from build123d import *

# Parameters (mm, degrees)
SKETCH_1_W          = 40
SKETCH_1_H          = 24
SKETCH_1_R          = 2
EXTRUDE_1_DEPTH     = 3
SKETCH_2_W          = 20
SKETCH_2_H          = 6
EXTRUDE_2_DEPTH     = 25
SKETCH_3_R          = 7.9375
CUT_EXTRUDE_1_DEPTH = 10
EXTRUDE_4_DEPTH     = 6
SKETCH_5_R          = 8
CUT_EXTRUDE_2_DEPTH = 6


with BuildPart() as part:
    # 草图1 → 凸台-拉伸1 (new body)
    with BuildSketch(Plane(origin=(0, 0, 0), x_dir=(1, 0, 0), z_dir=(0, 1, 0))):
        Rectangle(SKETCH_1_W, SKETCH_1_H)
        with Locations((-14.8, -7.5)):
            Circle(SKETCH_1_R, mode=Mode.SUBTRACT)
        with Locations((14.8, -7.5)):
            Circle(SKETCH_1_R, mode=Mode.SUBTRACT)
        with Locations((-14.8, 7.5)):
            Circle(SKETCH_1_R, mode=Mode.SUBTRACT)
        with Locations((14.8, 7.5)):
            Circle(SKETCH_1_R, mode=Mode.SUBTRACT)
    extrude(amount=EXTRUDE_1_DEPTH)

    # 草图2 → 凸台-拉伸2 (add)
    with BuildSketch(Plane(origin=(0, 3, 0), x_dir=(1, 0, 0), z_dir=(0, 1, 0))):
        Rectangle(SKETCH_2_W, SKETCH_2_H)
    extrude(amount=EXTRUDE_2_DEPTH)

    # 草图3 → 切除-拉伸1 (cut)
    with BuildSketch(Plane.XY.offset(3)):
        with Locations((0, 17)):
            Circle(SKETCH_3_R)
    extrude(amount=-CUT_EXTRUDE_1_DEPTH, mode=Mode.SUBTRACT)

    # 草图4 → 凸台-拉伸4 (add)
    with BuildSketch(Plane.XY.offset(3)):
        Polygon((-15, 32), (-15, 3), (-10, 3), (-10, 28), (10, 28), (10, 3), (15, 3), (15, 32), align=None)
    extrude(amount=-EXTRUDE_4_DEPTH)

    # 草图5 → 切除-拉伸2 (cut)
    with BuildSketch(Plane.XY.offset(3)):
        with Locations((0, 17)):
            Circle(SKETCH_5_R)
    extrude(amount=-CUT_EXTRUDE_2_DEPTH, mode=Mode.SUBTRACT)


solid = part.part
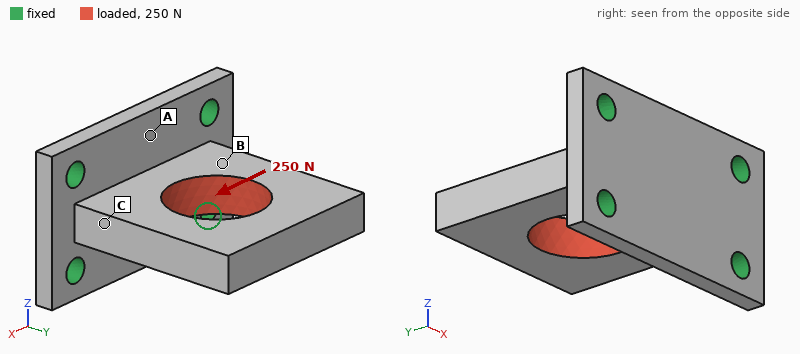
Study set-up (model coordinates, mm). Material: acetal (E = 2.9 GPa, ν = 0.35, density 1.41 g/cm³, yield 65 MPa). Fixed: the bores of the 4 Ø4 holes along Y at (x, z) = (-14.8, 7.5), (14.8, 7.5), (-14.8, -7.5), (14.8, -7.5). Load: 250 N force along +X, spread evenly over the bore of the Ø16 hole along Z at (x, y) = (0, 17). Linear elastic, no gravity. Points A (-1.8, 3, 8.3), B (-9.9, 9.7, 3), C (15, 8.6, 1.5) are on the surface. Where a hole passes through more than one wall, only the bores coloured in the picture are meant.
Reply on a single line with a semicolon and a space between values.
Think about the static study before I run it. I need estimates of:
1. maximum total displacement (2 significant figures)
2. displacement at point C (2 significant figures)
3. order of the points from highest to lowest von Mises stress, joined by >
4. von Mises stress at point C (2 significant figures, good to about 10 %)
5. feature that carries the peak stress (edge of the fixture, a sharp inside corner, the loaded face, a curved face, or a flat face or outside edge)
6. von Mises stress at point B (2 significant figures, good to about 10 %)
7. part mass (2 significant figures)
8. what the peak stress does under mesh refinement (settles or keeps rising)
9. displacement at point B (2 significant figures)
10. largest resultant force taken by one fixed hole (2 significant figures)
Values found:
0.16 mm; 0.048 mm; C > B > A; 6.1 MPa; edge of the fixture; 2.4 MPa; 9.5 g; keeps rising; 0.037 mm; 97 N
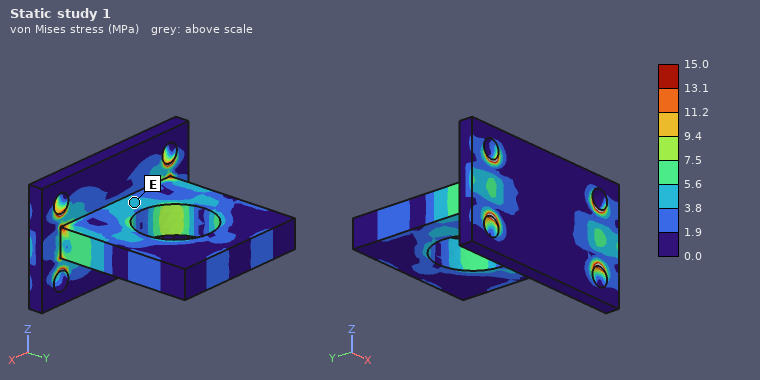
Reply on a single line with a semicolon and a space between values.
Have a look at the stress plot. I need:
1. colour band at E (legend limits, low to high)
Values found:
3.8 to 5.6 MPa
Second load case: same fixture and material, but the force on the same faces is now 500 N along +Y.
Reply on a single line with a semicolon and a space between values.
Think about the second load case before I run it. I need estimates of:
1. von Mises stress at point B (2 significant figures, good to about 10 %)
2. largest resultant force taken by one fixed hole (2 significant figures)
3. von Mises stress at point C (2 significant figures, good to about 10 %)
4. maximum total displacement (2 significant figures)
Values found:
3.8 MPa; 130 N; 6.2 MPa; 85 µm
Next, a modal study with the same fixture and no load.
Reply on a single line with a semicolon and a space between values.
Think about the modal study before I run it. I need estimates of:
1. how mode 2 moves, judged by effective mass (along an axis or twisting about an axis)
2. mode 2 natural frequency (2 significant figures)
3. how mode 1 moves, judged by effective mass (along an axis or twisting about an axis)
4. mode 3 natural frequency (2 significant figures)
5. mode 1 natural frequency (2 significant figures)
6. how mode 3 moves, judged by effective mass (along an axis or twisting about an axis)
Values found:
twisting about Y; 2600 Hz; along Z; 2900 Hz; 1100 Hz; along X
